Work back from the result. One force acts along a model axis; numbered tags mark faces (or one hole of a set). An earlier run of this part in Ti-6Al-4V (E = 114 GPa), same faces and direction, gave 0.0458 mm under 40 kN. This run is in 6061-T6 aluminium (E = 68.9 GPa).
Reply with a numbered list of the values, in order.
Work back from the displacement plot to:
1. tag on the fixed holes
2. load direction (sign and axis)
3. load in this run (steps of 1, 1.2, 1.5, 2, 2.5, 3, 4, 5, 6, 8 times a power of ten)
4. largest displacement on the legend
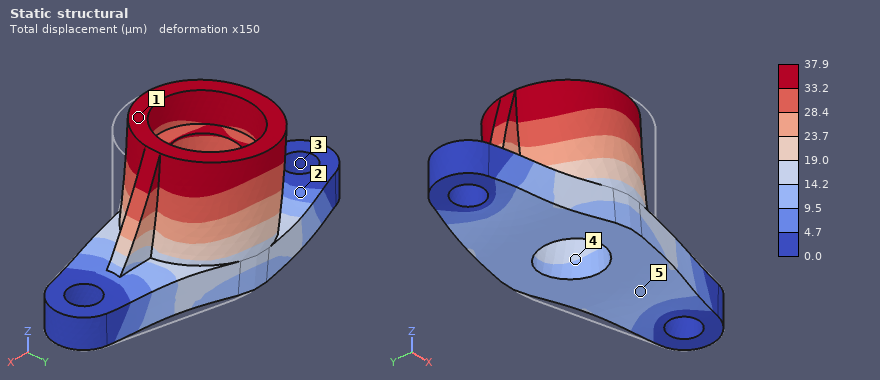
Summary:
1. 3
2. -X
3. 20 kN
4. 37.9 µm
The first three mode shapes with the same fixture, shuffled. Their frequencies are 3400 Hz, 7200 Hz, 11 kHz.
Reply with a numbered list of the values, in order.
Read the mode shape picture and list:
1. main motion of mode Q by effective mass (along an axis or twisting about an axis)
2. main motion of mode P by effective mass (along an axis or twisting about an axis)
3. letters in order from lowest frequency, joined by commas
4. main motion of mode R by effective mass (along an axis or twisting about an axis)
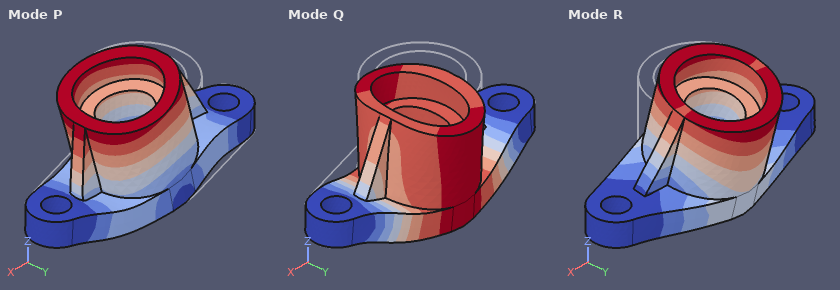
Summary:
1. along Z
2. along X
3. R, Q, P
4. along Y
